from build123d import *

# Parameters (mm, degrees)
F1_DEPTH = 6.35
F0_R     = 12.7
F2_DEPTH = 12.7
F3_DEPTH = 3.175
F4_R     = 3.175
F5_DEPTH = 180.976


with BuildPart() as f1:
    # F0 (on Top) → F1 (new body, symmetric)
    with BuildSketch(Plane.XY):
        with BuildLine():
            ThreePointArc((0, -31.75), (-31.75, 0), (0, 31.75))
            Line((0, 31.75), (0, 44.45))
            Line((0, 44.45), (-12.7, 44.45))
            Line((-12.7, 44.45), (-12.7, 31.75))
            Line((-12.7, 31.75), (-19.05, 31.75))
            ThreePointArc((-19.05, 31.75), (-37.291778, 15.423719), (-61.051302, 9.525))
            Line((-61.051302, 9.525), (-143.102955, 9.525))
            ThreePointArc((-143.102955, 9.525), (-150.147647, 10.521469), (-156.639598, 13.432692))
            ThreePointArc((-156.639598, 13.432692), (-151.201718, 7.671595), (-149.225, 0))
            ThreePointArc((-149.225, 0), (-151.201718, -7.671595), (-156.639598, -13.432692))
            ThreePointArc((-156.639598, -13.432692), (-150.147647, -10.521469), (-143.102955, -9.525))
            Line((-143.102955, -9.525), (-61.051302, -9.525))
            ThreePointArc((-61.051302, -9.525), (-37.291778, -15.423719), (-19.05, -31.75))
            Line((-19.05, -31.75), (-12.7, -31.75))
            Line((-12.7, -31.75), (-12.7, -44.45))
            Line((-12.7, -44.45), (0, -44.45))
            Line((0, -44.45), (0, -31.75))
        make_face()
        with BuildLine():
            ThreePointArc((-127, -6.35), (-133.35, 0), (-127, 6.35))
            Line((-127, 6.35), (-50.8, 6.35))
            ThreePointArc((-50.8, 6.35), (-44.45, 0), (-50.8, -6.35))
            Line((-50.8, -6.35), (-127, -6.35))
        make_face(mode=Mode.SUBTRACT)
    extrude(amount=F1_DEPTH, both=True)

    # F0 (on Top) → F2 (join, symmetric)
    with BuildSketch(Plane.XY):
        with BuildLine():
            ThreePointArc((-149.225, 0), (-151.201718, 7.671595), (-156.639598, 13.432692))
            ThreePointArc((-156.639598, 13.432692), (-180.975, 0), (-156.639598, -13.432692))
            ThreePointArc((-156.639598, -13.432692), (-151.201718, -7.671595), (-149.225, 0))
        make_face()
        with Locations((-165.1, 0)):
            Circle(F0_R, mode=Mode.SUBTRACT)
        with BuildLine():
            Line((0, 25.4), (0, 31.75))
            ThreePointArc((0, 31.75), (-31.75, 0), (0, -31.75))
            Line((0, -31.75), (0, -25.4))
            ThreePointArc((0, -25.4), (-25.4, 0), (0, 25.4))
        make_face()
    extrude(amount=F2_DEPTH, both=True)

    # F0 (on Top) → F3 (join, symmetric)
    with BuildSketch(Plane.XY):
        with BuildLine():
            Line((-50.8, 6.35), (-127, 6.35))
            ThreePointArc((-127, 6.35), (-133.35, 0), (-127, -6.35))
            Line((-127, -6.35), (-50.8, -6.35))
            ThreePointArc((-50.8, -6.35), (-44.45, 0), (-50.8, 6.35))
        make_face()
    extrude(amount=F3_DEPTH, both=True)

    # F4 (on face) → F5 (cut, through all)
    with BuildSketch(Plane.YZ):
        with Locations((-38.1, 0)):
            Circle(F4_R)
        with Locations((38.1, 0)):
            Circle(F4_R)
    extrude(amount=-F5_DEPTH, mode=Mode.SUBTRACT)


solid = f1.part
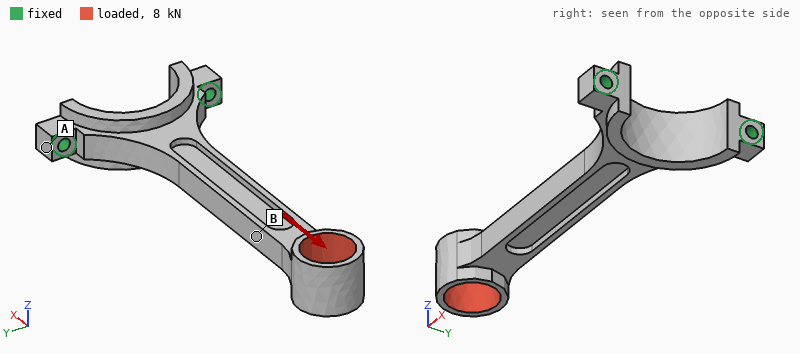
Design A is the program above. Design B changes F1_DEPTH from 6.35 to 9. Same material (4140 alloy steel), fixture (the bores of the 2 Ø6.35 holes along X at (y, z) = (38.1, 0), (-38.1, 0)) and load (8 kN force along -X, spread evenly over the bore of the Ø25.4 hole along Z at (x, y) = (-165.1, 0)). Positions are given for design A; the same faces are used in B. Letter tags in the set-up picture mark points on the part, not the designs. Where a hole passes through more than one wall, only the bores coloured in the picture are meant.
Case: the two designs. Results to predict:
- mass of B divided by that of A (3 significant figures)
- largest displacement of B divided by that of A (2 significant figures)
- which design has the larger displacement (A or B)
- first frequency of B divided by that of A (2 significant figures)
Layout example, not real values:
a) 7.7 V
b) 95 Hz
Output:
a) 1.19
b) 0.88
c) A
d) 1.4
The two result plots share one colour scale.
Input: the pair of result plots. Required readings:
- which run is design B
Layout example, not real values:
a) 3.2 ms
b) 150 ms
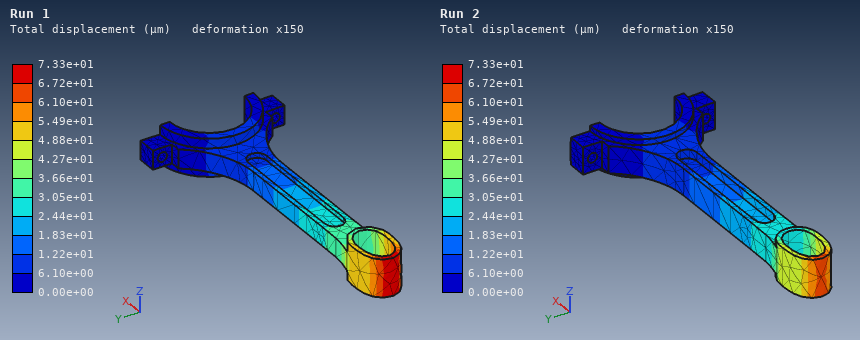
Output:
a) Run 2
